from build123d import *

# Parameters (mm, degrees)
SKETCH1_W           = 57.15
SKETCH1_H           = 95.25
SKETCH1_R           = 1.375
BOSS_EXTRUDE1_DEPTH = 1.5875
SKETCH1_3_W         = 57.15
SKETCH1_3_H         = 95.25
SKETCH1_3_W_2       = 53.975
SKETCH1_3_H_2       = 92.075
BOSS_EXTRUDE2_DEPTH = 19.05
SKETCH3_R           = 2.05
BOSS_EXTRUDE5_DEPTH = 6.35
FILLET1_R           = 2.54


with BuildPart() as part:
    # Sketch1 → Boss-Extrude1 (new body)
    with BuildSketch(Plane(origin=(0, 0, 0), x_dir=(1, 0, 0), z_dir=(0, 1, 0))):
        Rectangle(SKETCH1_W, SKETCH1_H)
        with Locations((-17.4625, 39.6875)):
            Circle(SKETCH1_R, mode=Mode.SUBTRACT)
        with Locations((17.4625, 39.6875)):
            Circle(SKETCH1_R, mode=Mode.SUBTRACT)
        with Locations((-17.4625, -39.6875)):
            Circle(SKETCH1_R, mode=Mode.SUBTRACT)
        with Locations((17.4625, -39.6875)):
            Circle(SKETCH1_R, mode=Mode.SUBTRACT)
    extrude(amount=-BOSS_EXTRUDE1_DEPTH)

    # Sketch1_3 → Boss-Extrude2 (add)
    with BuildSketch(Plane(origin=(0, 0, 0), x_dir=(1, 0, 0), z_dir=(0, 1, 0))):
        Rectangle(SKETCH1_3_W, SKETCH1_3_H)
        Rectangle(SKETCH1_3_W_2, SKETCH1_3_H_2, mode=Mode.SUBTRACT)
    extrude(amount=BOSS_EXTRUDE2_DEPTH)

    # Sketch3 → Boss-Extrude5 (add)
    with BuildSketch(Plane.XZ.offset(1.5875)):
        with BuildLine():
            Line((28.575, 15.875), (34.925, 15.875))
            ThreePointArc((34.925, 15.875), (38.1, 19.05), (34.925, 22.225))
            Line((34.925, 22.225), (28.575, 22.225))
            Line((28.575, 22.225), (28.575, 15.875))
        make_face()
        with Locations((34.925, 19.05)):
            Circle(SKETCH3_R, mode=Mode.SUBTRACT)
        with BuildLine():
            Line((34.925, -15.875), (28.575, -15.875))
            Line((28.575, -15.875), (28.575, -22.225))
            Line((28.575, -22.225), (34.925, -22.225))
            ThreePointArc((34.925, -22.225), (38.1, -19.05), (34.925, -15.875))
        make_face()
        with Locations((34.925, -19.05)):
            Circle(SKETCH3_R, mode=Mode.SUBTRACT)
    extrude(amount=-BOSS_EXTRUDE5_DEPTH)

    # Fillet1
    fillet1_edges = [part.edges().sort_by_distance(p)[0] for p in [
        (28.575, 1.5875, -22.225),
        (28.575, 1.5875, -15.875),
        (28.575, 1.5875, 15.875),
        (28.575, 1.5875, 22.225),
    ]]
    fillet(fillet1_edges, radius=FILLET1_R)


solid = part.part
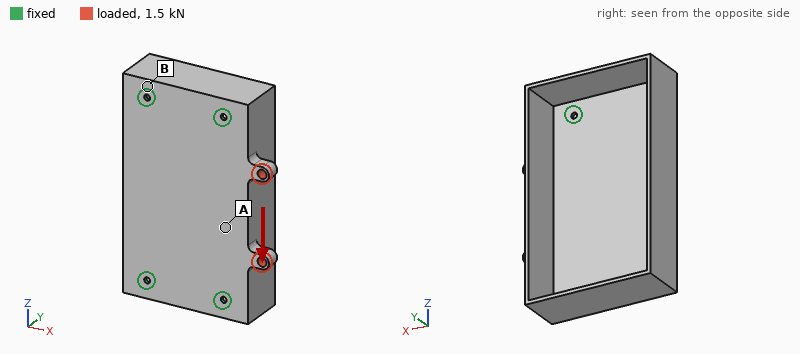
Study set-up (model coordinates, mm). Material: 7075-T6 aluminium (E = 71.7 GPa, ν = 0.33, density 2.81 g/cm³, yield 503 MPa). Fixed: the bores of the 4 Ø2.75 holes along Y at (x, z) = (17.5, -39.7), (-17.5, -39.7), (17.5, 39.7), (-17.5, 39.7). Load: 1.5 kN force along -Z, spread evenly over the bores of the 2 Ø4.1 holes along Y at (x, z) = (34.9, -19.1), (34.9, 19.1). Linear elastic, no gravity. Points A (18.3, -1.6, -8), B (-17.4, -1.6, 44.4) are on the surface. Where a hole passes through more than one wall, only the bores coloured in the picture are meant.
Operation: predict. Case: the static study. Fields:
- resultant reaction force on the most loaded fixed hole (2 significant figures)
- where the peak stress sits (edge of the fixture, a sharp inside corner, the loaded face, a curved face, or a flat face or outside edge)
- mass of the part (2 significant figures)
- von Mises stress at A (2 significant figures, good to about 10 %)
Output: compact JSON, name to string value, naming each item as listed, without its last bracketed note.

{"resultant reaction force on the most loaded fixed hole": "690 N", "where the peak stress sits": "a curved face", "mass of the part": "51 g", "von Mises stress at A": "25 MPa"}
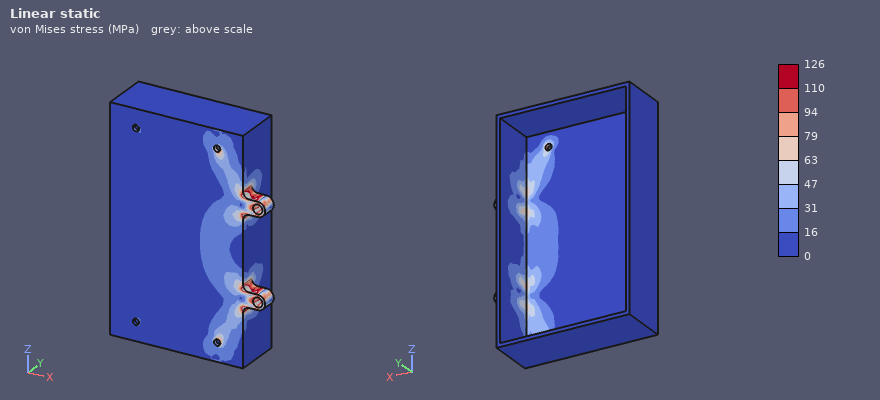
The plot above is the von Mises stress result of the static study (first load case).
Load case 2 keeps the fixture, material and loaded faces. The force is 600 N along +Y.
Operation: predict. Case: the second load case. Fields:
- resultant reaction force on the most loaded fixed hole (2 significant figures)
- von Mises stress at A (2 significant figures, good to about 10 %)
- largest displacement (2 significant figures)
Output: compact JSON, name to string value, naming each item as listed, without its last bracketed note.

{"resultant reaction force on the most loaded fixed hole": "500 N", "von Mises stress at A": "52 MPa", "largest displacement": "0.45 mm"}
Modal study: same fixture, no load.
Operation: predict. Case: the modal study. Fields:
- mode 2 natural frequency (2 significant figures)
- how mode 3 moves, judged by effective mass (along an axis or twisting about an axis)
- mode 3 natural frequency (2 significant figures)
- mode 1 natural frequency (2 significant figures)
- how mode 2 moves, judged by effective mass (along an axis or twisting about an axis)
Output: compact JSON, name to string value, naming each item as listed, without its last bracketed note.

{"mode 2 natural frequency": "2500 Hz", "how mode 3 moves, judged by effective mass": "along Y", "mode 3 natural frequency": "3300 Hz", "mode 1 natural frequency": "2000 Hz", "how mode 2 moves, judged by effective mass": "along X"}
